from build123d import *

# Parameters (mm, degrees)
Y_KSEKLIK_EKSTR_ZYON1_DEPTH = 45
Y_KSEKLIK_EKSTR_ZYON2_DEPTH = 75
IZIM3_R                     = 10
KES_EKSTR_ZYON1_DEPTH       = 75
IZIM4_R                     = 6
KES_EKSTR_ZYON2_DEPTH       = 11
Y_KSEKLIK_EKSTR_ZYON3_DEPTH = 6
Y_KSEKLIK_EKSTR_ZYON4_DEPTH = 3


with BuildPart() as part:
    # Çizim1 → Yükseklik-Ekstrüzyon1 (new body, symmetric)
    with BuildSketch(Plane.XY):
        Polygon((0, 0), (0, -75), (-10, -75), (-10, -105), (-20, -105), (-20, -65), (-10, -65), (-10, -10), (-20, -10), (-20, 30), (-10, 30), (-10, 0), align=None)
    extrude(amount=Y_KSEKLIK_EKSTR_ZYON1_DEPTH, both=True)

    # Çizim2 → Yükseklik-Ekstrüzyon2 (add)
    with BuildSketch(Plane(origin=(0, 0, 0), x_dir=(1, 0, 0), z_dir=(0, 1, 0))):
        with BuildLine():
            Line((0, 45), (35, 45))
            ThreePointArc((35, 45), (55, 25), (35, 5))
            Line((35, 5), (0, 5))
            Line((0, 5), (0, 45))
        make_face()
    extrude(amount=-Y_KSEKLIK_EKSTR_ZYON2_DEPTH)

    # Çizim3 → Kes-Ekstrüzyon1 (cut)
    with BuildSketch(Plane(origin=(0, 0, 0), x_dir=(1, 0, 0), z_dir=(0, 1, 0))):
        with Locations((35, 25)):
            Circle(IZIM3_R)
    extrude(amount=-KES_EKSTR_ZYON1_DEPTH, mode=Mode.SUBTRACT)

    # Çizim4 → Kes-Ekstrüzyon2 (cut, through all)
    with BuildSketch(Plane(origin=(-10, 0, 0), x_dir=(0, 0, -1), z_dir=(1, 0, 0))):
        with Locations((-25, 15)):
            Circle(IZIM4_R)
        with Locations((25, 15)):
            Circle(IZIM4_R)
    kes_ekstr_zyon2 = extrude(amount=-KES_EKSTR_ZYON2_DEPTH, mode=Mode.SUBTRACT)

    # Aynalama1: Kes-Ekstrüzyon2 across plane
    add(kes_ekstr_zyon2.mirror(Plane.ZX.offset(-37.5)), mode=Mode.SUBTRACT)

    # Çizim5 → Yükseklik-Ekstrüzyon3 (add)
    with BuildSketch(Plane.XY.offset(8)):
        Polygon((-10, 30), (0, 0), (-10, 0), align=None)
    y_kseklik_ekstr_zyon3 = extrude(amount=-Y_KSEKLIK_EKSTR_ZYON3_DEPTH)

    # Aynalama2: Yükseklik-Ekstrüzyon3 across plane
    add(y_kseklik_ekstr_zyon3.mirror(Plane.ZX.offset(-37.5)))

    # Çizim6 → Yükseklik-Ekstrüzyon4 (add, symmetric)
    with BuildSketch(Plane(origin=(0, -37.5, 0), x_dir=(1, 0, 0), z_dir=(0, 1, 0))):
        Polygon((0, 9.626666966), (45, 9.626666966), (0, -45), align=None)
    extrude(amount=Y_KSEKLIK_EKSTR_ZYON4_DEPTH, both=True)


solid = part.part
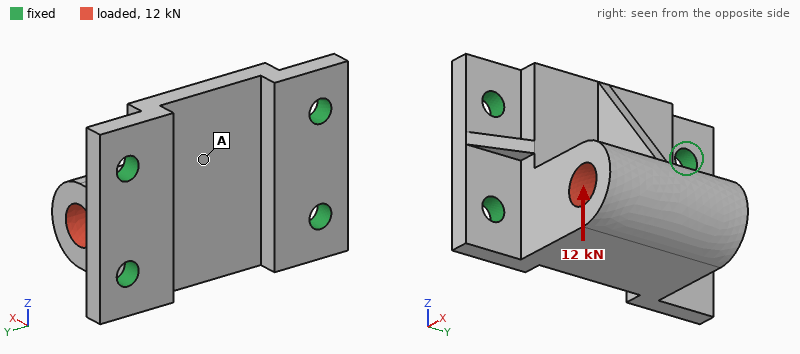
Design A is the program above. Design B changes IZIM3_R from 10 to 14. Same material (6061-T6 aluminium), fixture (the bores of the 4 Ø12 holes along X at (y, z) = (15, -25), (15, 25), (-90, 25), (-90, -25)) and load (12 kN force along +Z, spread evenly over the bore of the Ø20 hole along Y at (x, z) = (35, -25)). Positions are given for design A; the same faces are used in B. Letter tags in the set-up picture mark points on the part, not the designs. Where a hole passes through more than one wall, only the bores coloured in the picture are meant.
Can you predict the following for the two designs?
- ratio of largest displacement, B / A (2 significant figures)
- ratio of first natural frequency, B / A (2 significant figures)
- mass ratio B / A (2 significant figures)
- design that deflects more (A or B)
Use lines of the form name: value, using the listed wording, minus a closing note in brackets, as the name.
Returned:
ratio of largest displacement, B / A: 1.1
ratio of first natural frequency, B / A: 1.1
mass ratio B / A: 0.92
design that deflects more: B
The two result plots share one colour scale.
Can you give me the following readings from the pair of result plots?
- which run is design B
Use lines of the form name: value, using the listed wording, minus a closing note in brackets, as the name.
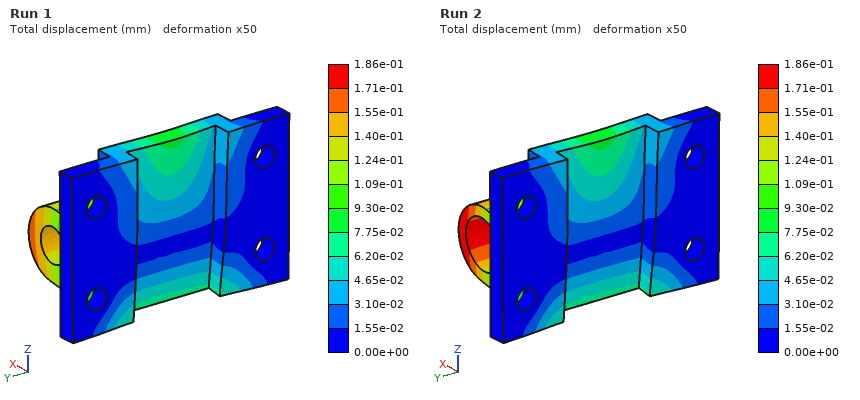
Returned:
which run is design B: Run 2
